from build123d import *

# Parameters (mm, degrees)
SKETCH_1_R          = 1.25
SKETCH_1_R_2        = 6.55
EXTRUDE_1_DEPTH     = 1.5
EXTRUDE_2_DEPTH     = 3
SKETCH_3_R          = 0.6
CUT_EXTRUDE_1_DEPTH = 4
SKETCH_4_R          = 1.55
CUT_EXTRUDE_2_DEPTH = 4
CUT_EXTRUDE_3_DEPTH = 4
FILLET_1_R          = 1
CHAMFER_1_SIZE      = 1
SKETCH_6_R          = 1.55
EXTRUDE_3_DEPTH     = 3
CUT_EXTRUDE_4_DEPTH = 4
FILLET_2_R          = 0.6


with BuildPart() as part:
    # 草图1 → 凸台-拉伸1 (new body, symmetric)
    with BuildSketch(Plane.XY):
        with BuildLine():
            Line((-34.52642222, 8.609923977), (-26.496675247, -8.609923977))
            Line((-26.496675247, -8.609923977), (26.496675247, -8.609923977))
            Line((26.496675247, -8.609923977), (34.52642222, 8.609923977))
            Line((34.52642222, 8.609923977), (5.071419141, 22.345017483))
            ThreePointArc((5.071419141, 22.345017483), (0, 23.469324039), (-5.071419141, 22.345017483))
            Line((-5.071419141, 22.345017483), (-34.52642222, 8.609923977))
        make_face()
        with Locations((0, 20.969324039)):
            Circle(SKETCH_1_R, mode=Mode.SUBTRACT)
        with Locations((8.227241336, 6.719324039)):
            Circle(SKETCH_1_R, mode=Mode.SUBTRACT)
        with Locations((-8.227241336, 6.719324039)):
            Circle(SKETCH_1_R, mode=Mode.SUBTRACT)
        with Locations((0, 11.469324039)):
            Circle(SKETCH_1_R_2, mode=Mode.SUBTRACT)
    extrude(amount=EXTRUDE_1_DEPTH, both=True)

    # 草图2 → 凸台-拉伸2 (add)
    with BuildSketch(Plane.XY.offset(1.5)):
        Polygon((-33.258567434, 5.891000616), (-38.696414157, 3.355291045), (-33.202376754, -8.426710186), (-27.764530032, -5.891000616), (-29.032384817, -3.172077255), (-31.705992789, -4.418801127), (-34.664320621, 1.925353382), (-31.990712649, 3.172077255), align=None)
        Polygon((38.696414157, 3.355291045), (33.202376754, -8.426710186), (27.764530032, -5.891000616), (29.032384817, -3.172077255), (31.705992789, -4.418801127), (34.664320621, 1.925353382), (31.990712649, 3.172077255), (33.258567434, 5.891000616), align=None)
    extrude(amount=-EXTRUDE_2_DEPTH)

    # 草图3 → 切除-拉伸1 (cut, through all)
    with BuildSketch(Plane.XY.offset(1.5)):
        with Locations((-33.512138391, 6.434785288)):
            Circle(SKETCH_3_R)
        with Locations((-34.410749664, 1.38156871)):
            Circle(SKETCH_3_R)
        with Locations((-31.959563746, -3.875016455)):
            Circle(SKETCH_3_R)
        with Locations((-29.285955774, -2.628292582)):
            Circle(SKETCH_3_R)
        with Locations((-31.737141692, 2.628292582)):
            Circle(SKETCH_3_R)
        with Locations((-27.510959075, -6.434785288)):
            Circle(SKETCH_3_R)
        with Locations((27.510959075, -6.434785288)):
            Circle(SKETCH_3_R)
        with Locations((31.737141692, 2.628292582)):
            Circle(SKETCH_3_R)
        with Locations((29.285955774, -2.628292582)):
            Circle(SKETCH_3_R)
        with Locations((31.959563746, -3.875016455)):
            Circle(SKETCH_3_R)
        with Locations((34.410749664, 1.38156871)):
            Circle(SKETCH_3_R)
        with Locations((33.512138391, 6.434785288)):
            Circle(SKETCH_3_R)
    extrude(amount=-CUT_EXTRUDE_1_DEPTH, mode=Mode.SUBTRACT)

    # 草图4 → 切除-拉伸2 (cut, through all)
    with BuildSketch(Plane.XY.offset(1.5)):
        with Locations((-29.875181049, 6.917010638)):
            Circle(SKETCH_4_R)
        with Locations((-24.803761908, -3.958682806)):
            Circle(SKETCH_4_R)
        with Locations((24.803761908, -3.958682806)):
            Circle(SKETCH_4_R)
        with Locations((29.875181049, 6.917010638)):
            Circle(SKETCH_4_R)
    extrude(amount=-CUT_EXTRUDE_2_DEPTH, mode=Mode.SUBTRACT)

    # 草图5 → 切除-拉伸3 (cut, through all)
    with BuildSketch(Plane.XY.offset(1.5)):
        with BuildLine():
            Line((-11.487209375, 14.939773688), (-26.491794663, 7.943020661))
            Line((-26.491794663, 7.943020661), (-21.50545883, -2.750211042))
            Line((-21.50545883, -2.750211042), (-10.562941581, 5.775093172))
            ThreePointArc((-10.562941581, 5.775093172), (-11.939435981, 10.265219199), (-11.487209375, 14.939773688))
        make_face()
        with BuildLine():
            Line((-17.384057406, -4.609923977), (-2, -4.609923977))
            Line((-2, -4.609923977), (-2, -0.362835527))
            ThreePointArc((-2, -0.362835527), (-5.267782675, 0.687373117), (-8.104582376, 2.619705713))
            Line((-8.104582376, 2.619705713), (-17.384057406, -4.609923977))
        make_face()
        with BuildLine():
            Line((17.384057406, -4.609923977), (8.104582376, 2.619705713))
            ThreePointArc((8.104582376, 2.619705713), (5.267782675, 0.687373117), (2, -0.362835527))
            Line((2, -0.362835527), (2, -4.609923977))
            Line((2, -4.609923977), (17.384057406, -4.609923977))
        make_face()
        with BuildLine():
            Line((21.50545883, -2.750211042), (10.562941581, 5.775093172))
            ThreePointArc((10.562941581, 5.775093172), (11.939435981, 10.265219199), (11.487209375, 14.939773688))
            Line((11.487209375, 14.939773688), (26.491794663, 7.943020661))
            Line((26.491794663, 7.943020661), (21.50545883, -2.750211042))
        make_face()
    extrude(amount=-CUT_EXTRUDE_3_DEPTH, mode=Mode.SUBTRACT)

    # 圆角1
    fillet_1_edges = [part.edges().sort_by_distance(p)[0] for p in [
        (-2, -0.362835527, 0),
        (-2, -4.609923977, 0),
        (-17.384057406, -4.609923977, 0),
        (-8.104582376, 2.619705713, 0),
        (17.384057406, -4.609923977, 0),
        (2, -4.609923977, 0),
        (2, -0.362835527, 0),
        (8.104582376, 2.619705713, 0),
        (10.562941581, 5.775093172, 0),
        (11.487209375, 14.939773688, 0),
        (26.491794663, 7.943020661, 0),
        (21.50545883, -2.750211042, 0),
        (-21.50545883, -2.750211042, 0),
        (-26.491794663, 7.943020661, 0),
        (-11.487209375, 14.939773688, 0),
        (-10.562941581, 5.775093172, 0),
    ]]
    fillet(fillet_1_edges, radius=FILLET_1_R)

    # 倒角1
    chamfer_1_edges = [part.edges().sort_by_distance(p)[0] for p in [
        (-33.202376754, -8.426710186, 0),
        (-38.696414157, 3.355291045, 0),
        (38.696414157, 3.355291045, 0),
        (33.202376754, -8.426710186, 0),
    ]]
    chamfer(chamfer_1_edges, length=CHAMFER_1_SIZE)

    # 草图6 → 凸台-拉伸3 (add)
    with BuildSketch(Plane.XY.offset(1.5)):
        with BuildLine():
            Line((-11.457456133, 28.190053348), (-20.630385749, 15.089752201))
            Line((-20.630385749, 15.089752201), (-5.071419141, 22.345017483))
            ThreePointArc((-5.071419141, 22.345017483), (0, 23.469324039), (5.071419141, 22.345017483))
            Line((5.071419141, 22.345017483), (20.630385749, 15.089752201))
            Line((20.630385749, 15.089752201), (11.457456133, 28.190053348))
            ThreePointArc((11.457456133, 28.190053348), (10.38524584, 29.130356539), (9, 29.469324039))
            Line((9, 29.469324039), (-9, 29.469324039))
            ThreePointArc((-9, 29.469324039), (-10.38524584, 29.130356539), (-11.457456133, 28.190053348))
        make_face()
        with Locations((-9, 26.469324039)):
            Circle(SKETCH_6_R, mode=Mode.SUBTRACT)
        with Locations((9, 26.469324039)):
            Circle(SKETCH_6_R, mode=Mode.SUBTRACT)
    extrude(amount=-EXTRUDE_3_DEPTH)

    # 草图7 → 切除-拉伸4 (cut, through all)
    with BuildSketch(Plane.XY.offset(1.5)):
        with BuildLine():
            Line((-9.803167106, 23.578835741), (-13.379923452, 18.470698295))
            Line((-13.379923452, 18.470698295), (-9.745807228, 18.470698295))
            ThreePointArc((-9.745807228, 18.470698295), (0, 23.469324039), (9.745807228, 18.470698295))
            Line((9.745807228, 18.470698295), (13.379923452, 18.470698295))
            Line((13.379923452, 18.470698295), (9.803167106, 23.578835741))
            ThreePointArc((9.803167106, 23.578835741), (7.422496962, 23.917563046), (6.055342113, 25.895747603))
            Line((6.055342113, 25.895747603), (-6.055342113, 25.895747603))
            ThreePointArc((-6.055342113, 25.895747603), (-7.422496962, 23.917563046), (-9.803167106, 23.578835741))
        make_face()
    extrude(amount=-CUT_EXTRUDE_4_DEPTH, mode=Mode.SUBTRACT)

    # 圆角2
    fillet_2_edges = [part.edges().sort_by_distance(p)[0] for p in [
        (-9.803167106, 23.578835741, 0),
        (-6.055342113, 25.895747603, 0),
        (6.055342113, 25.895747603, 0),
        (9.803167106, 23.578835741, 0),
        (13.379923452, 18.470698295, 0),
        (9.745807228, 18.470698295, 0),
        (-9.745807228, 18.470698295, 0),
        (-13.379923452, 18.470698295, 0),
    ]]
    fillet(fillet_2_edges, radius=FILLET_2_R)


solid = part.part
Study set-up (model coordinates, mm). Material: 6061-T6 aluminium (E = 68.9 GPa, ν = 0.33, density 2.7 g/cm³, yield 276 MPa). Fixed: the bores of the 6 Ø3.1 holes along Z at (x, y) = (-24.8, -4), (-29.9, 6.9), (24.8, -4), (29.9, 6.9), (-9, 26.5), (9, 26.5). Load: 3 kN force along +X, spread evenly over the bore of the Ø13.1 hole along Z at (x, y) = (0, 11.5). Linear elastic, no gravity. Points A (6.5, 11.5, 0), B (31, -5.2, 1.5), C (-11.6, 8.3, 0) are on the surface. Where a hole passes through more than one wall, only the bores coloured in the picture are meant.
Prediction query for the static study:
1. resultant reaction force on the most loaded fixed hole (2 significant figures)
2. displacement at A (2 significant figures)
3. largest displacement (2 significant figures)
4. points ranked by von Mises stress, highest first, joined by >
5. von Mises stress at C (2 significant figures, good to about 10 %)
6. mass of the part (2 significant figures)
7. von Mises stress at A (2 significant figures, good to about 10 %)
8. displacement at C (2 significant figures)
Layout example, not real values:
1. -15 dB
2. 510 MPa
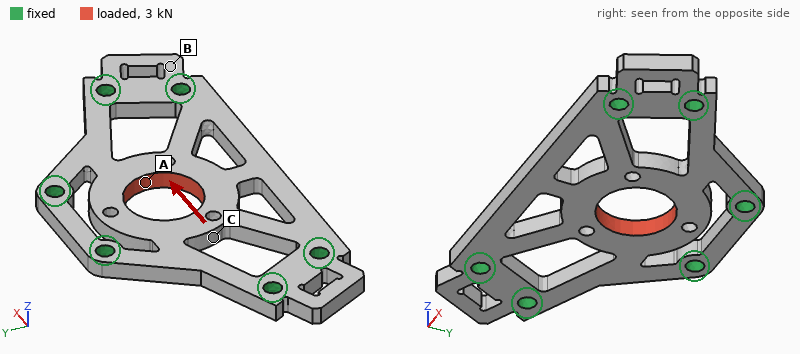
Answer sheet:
1. 800 N
2. 29 µm
3. 30 µm
4. C > A > B
5. 47 MPa
6. 10 g
7. 24 MPa
8. 29 µm
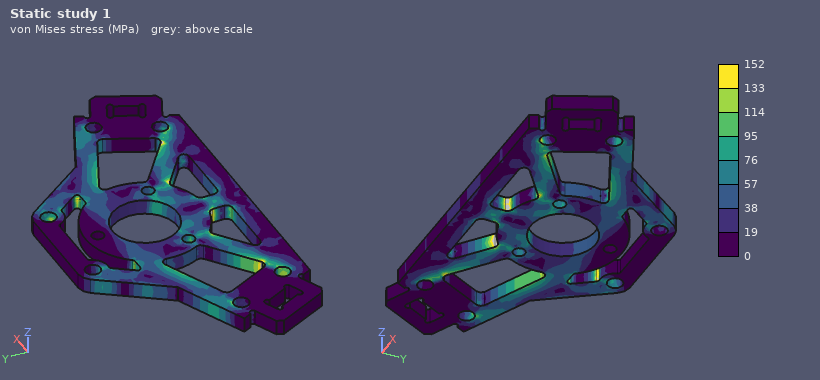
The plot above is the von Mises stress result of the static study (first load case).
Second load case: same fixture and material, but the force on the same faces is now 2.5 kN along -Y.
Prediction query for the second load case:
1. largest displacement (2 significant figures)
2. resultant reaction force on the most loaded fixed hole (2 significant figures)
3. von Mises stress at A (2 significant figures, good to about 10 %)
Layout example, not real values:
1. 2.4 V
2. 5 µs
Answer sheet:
1. 46 µm
2. 660 N
3. 56 MPa
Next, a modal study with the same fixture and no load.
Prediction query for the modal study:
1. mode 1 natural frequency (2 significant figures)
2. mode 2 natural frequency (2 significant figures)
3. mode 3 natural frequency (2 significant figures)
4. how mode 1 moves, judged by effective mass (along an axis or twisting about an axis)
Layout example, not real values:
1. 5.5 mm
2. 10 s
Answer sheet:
1. 6100 Hz
2. 9200 Hz
3. 14 kHz
4. along Z
